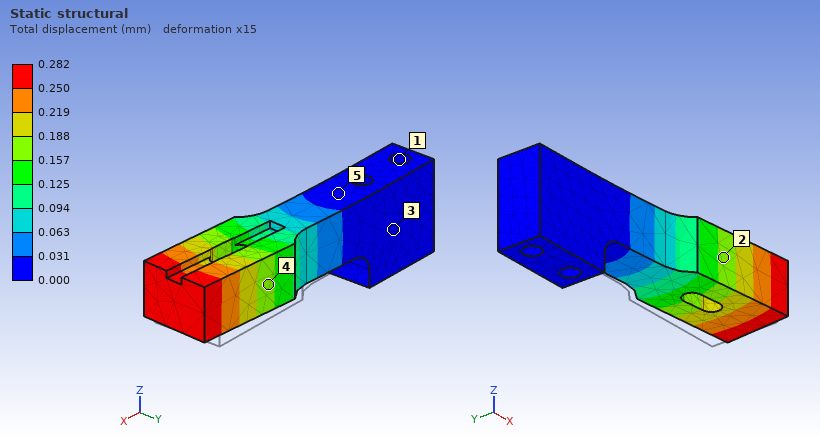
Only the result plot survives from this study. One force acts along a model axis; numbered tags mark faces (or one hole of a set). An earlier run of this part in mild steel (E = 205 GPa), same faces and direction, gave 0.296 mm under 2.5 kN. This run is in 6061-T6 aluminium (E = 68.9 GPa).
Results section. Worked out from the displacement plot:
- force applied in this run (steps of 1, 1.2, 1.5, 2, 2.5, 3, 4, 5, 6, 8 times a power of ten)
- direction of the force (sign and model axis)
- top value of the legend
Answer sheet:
800 N
-Y
0.282 mm
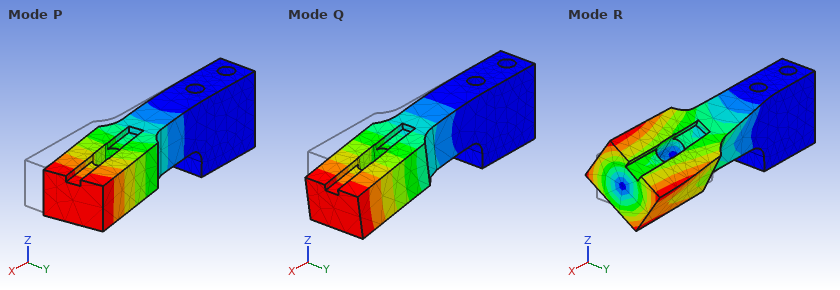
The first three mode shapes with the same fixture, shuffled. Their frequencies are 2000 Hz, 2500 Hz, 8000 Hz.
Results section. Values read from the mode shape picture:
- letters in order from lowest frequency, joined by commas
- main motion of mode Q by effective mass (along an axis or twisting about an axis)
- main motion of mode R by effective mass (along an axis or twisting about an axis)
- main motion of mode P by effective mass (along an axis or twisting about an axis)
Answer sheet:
P, Q, R
along Z
twisting about X
along Y
